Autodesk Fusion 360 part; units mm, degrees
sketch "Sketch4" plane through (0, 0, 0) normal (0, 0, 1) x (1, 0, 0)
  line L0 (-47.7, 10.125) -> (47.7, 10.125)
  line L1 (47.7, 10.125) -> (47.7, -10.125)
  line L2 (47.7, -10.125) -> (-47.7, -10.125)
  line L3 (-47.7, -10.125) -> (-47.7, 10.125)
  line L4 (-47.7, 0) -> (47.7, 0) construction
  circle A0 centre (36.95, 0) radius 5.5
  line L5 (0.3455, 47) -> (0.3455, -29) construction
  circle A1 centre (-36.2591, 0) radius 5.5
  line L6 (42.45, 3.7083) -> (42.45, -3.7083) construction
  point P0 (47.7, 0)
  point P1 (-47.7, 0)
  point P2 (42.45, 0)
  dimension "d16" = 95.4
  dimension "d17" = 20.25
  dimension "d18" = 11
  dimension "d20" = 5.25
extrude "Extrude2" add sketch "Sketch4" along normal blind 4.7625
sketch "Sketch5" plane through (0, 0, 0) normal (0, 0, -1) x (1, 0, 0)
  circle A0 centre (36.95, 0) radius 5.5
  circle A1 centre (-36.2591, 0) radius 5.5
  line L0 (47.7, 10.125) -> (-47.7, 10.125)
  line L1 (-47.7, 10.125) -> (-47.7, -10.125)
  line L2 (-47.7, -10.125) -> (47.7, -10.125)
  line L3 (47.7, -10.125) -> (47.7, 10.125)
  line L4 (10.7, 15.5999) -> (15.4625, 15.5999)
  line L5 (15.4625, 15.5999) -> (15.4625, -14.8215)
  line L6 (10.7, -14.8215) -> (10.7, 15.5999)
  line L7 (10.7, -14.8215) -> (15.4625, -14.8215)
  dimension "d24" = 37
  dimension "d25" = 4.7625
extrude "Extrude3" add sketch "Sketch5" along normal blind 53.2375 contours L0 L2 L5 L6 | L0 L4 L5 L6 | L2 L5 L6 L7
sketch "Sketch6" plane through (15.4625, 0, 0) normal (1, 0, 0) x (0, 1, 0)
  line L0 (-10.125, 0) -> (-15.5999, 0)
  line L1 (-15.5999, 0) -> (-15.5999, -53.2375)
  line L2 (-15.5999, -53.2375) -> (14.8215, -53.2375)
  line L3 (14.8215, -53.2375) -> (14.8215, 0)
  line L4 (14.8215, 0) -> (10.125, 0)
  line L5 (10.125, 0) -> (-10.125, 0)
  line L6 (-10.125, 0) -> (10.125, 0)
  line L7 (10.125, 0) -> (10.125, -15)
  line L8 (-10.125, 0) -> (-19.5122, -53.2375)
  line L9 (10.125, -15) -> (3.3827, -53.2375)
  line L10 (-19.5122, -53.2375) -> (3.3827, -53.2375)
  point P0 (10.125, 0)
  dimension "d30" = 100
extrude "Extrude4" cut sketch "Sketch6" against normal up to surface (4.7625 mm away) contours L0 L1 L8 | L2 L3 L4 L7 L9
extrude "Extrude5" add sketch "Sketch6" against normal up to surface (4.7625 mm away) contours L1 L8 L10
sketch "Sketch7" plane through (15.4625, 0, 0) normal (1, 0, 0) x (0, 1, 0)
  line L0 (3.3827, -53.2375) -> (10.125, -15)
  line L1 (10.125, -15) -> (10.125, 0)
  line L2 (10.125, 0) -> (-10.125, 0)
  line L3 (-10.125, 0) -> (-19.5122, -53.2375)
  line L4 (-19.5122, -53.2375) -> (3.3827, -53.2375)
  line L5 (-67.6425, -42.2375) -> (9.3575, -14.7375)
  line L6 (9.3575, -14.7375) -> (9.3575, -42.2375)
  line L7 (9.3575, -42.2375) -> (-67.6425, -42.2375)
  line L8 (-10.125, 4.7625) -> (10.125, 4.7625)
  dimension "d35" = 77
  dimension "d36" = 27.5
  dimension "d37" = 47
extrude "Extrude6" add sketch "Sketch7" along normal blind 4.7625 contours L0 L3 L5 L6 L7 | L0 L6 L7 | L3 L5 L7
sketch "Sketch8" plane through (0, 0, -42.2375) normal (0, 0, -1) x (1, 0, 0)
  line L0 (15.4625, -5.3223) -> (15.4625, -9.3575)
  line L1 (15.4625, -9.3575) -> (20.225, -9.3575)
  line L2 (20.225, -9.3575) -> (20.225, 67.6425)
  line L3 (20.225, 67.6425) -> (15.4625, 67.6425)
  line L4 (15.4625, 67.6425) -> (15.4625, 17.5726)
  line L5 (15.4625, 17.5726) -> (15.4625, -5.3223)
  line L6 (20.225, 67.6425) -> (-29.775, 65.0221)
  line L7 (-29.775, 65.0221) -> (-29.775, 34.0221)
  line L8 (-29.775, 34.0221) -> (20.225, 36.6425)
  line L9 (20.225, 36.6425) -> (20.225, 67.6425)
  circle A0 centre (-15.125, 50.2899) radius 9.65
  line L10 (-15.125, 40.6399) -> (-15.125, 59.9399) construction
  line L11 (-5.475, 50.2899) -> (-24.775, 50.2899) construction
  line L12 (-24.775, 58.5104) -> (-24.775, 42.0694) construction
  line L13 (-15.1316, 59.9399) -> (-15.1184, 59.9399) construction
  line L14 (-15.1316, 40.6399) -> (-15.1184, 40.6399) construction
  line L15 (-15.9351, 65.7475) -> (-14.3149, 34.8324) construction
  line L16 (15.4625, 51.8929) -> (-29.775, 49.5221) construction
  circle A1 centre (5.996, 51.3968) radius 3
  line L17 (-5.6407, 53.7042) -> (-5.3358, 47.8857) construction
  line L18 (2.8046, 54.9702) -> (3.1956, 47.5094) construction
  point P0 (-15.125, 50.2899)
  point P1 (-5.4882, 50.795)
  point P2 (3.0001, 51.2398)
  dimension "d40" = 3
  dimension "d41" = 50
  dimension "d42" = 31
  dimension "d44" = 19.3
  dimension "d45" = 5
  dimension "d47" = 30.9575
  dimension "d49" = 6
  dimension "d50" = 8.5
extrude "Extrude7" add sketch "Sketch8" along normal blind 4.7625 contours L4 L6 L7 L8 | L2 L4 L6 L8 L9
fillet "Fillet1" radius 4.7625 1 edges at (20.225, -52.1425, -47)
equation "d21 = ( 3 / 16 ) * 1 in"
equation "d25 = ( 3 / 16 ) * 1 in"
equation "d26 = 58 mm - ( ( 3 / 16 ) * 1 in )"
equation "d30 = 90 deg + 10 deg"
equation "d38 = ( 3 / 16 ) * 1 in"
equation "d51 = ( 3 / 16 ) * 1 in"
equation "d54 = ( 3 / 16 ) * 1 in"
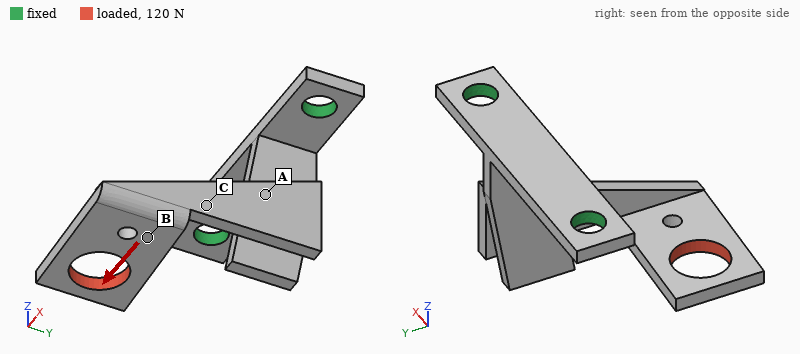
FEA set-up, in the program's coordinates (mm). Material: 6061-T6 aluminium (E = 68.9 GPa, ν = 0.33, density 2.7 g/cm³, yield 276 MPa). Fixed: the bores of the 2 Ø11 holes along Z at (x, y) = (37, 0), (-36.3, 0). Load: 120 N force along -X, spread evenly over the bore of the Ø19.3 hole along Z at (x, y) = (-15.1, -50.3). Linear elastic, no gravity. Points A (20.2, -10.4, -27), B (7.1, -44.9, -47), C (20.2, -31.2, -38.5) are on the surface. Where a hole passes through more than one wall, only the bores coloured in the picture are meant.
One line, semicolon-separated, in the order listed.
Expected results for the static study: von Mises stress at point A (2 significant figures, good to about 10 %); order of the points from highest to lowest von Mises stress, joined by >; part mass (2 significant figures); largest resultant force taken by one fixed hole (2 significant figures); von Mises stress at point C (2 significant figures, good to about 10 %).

26 MPa; C > A > B; 67 g; 170 N; 54 MPa
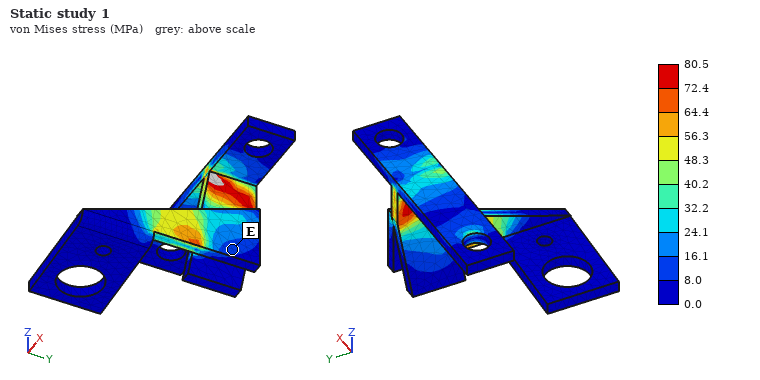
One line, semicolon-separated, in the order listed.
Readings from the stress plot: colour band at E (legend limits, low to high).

8.0 to 16.1 MPa
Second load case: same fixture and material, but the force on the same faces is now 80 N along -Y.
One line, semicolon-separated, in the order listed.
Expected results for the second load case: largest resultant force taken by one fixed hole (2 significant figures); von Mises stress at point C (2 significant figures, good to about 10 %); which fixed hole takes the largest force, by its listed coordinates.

53 N; 54 MPa; (-36.3, 0)
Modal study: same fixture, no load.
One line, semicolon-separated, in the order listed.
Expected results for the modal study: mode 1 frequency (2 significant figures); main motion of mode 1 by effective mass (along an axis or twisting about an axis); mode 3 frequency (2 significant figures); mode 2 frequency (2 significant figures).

370 Hz; along X; 880 Hz; 480 Hz
